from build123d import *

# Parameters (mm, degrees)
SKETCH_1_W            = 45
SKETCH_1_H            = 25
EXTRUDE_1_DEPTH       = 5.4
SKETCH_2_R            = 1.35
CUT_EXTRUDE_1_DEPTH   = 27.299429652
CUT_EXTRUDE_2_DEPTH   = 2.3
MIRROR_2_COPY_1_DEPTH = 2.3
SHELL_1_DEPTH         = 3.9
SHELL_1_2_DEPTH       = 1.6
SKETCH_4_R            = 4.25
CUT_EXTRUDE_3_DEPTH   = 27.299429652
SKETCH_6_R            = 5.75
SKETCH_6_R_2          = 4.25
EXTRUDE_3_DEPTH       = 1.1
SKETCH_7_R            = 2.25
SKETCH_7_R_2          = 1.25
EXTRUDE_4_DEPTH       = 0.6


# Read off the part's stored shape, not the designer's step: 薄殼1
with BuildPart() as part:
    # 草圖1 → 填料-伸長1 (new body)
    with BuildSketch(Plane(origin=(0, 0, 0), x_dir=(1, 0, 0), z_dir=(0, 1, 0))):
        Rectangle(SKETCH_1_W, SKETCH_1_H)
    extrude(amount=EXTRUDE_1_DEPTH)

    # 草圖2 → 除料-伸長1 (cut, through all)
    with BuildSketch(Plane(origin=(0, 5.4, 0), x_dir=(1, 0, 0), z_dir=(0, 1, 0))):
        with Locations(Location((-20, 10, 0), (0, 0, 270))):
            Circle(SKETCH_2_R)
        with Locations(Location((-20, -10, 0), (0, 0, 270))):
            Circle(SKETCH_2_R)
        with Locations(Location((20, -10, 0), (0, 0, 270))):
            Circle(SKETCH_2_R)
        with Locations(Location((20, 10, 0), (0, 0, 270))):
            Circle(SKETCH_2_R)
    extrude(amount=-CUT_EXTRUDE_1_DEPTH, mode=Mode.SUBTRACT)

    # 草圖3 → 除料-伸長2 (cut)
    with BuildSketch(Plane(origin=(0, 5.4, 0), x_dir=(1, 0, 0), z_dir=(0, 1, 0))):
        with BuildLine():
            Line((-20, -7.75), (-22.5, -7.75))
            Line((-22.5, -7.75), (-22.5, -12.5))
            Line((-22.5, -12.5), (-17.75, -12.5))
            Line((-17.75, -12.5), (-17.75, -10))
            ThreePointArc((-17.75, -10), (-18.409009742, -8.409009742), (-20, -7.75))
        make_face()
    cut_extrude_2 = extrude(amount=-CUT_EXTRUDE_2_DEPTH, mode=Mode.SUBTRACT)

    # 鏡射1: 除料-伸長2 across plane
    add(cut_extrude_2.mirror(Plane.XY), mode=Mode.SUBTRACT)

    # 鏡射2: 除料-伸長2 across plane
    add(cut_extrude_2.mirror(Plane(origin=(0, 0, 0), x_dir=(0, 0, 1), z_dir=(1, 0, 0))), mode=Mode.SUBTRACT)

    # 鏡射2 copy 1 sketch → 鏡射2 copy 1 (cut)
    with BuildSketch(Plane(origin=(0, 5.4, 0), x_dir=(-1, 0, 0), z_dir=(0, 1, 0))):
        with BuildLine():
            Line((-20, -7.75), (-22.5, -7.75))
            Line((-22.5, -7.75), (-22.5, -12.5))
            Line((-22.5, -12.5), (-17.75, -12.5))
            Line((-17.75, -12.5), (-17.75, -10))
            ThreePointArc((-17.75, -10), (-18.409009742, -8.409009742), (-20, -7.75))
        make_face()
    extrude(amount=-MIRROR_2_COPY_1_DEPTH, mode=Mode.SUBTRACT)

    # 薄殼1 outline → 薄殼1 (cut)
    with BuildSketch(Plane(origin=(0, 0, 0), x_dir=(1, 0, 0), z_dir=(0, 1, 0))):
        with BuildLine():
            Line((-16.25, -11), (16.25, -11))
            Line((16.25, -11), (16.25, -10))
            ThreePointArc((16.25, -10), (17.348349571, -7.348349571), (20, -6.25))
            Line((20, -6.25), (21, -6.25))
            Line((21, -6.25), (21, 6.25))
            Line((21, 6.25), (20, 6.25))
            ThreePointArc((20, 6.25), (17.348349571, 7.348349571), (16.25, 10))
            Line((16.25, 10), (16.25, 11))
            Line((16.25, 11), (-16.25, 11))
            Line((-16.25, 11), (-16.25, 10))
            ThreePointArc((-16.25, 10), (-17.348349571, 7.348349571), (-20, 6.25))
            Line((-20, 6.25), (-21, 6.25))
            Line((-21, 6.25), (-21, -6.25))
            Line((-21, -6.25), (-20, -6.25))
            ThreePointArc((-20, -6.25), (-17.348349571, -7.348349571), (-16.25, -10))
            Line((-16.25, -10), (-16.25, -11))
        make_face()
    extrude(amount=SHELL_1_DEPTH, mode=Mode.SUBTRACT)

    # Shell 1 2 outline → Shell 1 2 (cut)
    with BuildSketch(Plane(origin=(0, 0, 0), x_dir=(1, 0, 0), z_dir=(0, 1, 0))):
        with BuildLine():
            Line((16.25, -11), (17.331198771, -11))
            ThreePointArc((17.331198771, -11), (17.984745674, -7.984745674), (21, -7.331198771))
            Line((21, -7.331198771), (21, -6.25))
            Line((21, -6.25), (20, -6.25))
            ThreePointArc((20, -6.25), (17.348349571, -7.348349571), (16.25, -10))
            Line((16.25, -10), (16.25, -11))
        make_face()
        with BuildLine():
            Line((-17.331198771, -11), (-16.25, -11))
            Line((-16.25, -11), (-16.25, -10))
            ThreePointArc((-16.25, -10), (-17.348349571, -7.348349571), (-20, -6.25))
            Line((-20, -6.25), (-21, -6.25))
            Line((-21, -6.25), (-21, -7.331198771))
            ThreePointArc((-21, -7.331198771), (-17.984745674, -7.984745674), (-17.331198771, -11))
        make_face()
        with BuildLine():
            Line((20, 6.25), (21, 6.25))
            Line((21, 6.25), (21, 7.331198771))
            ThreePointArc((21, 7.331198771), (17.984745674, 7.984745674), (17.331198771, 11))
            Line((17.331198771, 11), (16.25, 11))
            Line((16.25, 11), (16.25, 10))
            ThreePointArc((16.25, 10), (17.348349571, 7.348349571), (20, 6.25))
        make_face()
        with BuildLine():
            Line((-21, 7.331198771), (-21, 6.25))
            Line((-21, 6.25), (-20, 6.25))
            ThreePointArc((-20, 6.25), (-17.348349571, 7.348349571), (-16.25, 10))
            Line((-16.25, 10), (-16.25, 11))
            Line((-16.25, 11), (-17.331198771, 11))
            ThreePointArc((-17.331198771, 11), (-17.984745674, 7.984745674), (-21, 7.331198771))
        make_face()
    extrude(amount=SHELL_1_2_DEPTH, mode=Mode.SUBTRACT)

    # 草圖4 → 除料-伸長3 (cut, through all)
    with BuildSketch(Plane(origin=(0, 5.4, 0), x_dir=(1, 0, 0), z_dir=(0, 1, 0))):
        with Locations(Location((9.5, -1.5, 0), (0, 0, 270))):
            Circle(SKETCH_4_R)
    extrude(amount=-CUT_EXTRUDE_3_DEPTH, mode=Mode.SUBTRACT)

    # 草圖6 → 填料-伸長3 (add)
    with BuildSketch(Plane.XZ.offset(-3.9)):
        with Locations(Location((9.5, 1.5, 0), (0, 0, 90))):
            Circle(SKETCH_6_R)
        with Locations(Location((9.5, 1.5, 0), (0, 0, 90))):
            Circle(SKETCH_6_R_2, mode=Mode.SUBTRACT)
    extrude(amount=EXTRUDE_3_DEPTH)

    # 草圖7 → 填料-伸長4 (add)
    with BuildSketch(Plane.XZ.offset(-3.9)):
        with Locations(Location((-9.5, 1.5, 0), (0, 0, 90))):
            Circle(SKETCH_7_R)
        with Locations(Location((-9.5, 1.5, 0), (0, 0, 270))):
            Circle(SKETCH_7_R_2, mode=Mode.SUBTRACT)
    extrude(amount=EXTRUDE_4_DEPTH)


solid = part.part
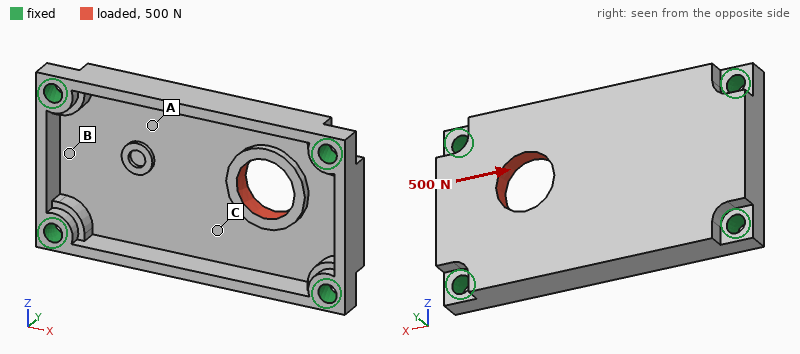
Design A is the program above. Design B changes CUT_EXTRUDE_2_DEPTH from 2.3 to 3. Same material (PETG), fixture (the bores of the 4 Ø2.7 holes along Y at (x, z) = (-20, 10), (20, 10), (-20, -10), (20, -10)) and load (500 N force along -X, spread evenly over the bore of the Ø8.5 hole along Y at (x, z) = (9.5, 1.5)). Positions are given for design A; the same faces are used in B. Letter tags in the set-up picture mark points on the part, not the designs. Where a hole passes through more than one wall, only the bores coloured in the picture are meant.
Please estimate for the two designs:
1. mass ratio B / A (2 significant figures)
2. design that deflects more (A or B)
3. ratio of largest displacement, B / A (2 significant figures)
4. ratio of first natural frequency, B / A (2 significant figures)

0.99
B
1.1
0.99
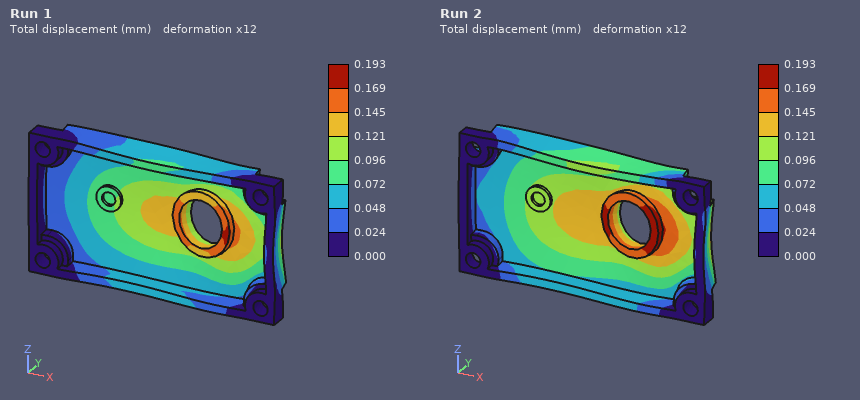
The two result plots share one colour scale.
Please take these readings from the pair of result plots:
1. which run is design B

Run 2
